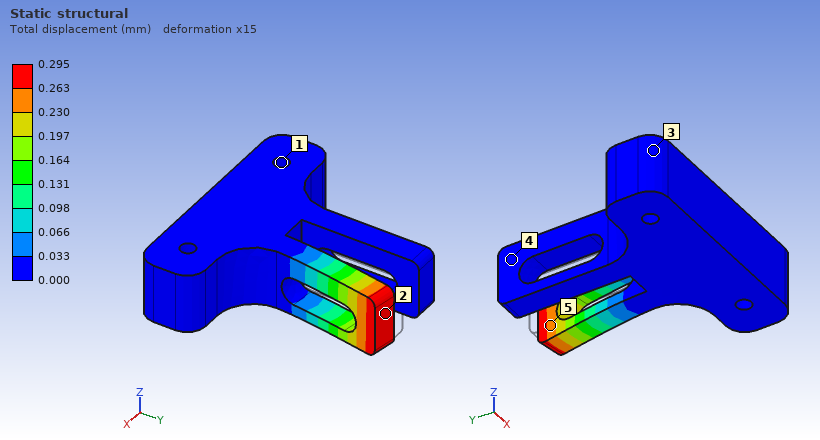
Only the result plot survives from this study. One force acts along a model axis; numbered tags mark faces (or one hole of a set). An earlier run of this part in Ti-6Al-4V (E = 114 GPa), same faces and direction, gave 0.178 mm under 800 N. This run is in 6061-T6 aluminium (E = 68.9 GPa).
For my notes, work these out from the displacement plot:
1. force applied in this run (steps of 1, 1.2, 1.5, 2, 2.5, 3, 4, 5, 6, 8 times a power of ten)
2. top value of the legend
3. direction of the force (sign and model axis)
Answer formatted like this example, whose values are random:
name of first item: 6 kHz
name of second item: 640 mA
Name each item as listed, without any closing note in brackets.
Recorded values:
force applied in this run: 800 N
top value of the legend: 0.295 mm
direction of the force: +X
